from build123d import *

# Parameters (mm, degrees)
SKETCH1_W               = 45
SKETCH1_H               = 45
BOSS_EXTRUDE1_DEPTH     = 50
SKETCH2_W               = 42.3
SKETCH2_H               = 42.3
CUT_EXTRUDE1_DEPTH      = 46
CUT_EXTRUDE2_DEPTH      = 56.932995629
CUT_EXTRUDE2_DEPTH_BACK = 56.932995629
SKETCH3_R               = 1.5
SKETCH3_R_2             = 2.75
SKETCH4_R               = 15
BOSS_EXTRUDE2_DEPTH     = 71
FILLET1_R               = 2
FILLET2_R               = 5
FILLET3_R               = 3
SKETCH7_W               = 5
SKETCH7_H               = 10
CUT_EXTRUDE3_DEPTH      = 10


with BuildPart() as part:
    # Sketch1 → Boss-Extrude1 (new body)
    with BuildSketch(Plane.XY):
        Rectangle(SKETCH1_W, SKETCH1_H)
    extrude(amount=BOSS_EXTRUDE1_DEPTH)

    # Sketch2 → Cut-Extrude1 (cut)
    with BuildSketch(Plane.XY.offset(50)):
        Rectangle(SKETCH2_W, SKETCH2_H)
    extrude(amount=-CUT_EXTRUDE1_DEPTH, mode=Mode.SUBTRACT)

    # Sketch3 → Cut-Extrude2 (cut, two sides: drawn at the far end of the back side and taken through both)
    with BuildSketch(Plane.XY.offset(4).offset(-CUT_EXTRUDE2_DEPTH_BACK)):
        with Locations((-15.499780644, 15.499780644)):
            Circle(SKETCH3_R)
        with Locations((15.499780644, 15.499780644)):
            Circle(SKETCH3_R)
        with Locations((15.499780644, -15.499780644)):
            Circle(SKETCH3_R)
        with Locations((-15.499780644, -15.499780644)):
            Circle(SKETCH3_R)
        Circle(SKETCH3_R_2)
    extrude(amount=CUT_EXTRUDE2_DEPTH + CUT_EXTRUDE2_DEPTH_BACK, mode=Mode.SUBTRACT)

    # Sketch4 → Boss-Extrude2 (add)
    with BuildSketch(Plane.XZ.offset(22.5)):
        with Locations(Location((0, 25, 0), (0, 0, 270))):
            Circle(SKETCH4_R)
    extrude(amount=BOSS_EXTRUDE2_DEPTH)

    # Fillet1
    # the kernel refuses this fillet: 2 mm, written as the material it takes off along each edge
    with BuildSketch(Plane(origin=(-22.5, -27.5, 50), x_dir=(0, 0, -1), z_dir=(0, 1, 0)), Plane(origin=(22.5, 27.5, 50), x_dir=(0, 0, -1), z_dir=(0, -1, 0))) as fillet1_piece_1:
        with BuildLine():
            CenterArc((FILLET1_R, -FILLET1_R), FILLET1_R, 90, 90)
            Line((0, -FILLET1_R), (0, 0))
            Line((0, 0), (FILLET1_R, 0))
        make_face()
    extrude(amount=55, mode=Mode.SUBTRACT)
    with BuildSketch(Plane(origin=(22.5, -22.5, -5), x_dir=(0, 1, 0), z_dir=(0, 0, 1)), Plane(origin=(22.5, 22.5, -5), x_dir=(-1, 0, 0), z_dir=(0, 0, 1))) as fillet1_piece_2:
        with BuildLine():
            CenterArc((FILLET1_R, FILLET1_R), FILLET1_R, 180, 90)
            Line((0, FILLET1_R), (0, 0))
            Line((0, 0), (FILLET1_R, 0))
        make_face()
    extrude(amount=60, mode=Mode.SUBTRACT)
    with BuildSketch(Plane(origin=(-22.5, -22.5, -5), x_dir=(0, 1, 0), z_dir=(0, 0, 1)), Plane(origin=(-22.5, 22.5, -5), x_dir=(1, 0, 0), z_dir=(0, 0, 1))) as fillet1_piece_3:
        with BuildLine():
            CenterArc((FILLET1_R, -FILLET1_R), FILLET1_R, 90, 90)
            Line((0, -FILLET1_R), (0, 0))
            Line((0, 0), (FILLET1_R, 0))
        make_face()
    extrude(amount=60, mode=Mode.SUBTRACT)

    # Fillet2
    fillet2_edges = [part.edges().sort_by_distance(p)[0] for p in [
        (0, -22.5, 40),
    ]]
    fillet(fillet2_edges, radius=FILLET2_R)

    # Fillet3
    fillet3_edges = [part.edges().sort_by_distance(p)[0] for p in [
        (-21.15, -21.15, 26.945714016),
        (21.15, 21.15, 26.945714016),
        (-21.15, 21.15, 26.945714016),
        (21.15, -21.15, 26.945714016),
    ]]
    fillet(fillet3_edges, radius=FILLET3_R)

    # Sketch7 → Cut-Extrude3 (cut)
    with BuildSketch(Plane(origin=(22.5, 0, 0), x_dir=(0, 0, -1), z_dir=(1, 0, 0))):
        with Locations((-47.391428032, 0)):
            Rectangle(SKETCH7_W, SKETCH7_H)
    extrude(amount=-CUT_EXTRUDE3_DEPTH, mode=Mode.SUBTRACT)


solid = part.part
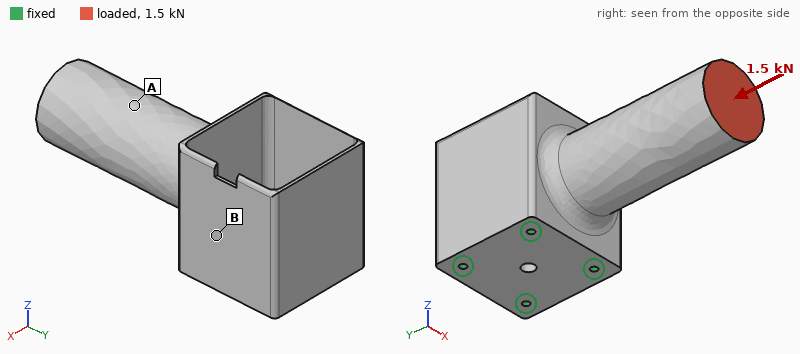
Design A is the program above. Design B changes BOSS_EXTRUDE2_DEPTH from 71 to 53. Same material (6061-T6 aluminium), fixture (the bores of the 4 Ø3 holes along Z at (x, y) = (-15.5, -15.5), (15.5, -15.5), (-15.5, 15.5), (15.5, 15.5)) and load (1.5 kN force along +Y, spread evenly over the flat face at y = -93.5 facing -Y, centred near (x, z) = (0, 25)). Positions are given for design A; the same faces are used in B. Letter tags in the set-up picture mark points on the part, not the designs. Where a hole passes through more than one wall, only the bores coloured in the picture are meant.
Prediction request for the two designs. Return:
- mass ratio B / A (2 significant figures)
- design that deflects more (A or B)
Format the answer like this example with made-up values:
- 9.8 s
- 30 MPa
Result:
- 0.82
- A
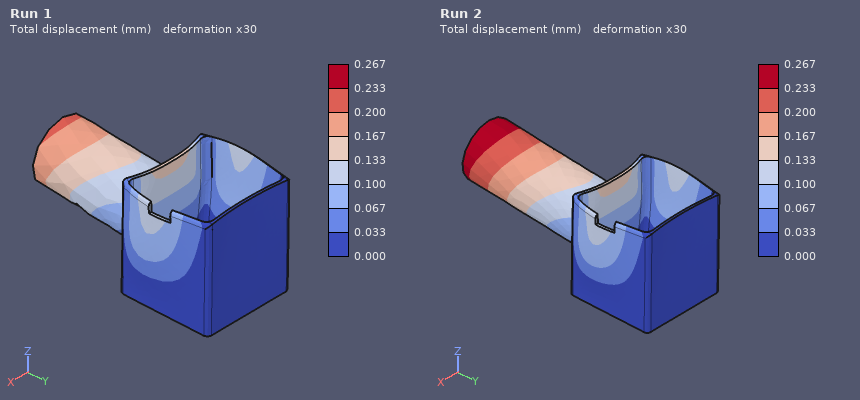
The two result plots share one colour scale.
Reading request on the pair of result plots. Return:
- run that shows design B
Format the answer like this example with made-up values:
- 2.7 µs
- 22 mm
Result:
- Run 1
